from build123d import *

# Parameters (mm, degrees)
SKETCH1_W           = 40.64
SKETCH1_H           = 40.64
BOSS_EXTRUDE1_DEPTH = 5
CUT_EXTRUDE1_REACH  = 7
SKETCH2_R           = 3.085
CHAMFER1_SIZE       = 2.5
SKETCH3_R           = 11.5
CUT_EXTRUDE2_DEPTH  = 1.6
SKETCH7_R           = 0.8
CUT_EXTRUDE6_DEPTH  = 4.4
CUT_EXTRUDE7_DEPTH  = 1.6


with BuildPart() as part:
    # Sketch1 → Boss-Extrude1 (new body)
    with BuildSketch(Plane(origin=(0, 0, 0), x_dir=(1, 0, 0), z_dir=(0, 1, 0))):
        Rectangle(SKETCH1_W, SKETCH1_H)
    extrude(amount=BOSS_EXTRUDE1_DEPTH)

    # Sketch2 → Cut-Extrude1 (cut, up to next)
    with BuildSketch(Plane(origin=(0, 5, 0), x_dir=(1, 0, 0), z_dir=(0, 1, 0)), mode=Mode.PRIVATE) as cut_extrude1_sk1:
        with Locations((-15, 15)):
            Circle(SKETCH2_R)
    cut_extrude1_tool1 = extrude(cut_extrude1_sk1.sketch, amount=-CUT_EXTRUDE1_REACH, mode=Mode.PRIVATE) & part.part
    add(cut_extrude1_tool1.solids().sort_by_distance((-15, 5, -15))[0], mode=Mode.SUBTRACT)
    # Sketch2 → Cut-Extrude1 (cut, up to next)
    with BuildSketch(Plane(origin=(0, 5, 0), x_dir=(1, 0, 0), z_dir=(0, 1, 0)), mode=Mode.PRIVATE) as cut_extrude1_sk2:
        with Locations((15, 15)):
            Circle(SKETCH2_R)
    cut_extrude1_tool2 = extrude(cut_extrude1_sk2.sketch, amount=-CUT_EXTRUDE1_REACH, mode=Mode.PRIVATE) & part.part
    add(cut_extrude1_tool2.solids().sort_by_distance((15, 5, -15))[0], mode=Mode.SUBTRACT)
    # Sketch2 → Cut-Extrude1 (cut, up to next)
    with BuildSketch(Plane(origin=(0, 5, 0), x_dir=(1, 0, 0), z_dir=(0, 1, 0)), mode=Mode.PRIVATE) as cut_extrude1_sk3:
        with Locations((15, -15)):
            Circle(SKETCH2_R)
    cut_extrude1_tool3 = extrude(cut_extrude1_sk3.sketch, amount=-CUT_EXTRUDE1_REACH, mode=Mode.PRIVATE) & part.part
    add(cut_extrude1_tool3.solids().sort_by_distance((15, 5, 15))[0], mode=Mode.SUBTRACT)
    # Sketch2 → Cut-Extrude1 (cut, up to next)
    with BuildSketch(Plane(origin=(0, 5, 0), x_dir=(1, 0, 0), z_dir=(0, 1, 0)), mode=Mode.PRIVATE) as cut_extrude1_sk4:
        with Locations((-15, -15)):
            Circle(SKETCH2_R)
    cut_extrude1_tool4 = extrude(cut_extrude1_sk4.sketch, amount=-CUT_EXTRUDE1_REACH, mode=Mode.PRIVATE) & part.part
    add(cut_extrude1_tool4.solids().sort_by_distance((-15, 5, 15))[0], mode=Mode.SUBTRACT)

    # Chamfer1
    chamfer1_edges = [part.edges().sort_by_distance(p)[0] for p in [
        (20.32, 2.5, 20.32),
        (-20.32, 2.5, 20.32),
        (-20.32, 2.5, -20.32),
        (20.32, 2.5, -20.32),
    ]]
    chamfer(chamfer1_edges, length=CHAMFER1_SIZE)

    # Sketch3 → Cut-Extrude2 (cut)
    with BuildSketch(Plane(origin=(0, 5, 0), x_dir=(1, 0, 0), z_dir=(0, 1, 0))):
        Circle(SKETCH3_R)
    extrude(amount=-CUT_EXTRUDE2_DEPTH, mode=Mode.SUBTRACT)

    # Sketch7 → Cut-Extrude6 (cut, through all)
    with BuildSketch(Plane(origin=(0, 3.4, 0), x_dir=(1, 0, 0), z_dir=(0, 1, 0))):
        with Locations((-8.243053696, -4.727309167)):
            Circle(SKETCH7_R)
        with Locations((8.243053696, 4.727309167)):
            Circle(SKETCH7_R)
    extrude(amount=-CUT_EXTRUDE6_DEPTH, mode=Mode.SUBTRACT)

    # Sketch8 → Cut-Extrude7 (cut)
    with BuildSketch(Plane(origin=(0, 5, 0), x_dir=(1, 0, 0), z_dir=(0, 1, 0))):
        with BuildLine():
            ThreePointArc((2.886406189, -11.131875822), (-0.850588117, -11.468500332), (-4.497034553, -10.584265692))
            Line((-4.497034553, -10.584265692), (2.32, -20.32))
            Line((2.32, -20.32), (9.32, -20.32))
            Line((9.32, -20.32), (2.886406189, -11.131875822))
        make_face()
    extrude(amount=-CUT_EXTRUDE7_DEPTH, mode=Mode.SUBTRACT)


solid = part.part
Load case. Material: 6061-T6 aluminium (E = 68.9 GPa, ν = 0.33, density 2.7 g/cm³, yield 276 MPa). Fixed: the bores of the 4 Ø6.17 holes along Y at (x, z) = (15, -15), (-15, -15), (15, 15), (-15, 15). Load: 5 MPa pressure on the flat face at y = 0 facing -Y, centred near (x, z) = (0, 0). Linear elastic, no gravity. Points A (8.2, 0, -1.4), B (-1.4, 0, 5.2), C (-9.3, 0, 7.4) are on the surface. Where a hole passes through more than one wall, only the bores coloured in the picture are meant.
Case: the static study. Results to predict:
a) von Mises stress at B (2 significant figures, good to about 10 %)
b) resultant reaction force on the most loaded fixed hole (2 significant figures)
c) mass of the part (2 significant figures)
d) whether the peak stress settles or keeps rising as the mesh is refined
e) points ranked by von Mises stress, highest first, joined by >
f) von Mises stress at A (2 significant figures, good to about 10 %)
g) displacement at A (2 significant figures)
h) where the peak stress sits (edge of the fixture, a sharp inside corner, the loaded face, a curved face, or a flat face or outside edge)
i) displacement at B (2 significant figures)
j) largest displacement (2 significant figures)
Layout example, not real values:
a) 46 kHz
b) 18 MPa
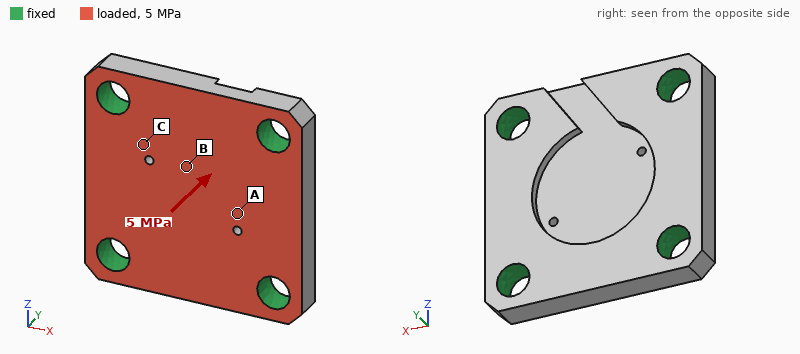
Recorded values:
a) 55 MPa
b) 2.0 kN
c) 18 g
d) keeps rising
e) B > A > C
f) 42 MPa
g) 28 µm
h) edge of the fixture
i) 35 µm
j) 39 µm
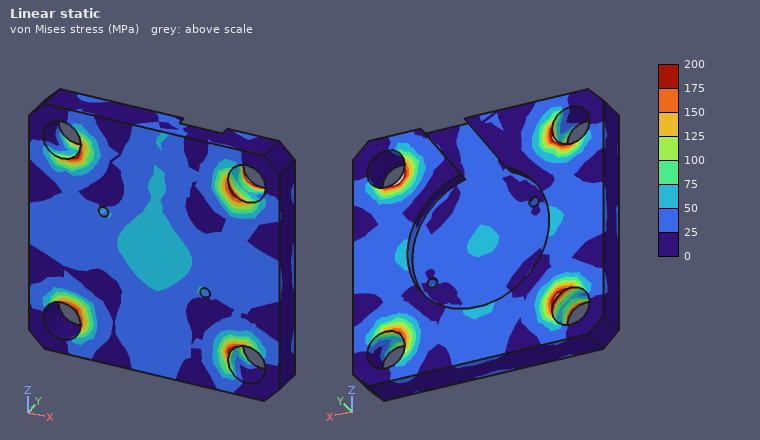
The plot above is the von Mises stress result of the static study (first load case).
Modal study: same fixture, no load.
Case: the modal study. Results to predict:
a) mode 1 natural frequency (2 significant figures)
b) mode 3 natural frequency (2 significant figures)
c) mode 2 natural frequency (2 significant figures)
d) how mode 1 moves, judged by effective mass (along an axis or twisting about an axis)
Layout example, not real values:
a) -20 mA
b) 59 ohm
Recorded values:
a) 23 kHz
b) 33 kHz
c) 33 kHz
d) along Y
